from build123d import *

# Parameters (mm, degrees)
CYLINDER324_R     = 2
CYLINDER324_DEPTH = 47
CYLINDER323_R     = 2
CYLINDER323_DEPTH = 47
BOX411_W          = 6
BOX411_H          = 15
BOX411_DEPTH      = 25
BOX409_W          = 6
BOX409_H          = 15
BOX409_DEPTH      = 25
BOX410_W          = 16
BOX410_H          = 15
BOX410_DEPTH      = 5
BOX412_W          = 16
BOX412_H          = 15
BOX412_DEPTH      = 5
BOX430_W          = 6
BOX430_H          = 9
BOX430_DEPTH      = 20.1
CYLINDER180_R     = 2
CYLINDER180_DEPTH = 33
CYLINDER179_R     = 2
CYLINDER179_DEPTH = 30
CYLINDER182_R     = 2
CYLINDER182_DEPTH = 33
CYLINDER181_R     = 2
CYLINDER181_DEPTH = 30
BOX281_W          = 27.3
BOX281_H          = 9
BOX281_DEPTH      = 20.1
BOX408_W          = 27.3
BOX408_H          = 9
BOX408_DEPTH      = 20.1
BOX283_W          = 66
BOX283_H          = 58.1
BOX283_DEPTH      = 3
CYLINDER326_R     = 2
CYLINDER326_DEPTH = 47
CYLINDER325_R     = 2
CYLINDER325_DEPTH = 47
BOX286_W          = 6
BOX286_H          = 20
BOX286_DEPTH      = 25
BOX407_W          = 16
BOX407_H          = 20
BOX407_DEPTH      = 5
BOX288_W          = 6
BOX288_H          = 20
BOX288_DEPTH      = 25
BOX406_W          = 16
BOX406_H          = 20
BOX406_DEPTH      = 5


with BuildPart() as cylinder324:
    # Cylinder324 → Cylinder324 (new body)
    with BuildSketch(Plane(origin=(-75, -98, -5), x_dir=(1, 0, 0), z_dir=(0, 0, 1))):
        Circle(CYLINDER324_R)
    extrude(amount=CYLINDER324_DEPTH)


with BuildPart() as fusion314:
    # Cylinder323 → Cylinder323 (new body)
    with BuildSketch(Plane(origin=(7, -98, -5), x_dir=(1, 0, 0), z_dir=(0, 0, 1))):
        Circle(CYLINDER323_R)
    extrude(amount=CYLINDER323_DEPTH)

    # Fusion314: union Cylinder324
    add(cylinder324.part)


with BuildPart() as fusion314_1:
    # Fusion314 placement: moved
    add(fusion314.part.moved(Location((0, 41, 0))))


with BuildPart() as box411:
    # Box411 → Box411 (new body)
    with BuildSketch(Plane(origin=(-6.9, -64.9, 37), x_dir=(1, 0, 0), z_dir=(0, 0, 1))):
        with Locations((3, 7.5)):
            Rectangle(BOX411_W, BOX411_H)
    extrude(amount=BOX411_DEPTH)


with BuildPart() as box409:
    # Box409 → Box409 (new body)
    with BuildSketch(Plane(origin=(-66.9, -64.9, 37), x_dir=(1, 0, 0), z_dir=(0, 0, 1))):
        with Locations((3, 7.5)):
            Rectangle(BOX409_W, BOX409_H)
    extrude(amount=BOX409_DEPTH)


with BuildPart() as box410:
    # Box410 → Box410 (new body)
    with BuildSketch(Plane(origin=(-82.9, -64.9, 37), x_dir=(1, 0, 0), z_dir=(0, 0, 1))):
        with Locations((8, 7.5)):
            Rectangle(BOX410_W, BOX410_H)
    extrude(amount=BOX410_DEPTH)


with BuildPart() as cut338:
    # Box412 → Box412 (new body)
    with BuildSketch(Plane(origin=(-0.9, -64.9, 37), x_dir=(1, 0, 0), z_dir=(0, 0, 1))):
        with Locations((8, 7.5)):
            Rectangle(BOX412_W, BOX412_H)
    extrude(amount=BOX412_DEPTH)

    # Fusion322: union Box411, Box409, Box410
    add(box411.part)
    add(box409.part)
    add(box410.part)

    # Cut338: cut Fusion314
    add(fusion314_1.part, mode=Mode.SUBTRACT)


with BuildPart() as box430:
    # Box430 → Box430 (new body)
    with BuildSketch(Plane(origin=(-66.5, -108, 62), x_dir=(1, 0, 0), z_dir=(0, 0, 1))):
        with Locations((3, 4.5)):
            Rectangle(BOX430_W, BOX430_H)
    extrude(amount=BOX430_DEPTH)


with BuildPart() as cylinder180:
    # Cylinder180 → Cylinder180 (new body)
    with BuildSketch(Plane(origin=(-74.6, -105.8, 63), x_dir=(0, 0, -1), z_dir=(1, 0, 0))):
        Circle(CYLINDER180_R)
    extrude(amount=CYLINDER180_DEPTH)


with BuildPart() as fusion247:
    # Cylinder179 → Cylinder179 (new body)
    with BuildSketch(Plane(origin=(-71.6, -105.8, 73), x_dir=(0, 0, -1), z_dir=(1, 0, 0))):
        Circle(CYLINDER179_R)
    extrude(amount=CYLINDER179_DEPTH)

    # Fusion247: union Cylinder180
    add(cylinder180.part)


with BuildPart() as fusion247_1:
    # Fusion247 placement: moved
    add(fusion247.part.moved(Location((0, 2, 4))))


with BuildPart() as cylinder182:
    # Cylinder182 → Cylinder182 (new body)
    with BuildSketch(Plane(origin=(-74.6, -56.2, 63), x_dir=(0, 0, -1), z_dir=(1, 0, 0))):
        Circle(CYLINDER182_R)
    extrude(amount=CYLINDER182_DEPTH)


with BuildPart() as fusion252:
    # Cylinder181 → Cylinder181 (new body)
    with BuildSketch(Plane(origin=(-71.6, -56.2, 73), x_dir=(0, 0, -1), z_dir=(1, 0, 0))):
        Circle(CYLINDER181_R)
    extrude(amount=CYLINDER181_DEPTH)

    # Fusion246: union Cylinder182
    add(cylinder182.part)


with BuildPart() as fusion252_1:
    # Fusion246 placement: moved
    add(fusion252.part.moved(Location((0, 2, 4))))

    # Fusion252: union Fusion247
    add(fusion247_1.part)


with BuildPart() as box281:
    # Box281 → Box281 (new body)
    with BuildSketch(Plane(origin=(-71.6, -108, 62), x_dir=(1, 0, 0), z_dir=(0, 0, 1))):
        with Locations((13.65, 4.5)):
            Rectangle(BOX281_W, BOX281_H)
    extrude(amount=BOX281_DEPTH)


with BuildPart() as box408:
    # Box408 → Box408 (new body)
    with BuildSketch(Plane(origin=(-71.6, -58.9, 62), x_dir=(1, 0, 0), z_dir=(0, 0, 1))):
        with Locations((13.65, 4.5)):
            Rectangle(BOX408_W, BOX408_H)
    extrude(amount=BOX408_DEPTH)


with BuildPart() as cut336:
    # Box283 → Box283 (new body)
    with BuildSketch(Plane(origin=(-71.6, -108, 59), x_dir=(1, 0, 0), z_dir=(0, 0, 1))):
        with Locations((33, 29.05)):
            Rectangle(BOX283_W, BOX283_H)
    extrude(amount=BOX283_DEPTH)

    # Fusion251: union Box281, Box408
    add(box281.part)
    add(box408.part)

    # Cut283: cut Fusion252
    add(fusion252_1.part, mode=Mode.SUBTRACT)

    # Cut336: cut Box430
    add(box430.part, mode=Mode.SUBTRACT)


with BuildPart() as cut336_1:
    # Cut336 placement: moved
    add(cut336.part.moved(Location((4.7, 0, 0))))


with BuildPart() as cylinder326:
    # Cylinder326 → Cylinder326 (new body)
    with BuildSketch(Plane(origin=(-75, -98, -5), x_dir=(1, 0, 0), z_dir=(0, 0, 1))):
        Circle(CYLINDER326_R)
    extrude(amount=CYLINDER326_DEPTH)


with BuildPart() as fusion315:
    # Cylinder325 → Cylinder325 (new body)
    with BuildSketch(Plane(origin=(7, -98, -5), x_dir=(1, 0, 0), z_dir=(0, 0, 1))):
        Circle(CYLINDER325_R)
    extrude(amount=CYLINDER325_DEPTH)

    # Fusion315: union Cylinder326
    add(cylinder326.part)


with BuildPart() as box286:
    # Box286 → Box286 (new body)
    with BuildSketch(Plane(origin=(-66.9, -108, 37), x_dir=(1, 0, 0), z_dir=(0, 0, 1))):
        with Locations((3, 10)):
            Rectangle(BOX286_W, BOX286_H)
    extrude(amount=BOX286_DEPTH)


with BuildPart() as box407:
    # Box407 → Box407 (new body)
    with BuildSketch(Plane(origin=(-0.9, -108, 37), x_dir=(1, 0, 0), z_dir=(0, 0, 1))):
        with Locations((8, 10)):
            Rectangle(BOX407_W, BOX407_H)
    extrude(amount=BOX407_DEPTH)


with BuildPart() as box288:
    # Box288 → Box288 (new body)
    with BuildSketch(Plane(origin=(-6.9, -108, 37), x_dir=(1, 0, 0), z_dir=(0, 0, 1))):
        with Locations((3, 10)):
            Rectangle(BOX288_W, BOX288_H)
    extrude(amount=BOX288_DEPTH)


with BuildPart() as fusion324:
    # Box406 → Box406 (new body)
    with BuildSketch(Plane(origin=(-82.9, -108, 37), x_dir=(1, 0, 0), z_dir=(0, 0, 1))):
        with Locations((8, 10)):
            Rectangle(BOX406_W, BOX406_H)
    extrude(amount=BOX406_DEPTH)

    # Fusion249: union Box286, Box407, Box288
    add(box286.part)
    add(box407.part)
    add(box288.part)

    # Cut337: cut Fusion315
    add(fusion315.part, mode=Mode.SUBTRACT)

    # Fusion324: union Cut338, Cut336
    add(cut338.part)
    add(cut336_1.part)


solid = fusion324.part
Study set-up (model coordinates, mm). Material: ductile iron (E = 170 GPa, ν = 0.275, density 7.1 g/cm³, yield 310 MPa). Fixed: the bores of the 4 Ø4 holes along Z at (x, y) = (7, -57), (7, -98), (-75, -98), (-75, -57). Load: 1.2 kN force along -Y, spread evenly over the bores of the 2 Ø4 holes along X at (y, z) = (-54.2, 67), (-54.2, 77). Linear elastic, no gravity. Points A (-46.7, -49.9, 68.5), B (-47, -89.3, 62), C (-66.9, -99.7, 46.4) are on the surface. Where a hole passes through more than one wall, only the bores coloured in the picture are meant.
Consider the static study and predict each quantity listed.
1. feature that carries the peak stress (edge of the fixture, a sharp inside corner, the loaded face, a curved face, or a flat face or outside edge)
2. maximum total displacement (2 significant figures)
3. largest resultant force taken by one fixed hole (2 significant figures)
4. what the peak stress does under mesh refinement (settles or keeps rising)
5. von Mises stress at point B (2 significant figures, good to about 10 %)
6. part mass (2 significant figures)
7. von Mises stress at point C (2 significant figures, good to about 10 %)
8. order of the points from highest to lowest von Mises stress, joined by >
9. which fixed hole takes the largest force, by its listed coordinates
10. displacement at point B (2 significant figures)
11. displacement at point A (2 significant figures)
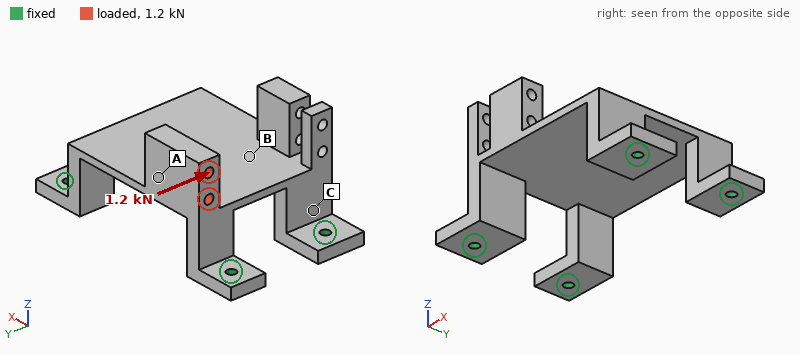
edge of the fixture
0.12 mm
770 N
keeps rising
28 MPa
240 g
46 MPa
C > B > A
(-75, -98)
0.035 mm
0.075 mm
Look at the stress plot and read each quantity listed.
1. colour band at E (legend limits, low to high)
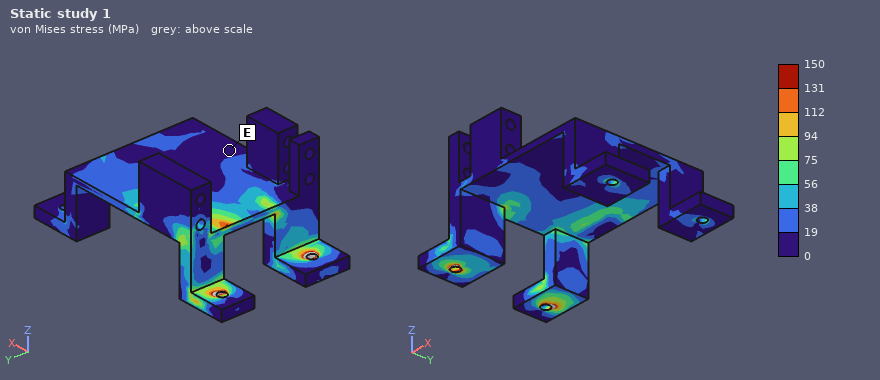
0 to 19 MPa
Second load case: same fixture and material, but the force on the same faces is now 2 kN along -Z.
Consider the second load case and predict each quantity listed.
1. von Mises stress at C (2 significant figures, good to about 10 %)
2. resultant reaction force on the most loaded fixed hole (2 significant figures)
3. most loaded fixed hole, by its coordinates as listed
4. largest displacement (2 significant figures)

21 MPa
1.9 kN
(-75, -57)
0.13 mm
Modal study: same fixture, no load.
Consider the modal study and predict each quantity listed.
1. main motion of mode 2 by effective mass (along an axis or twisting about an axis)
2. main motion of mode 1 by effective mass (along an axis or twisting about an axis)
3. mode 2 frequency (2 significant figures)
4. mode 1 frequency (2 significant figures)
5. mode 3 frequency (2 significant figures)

along X
along Y
2300 Hz
2200 Hz
3300 Hz
